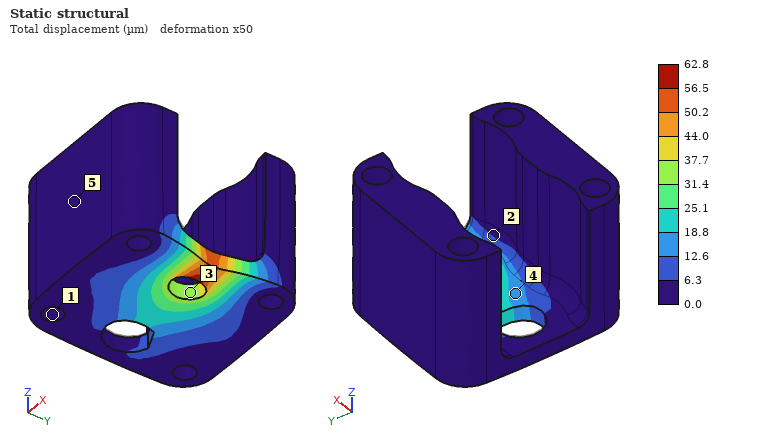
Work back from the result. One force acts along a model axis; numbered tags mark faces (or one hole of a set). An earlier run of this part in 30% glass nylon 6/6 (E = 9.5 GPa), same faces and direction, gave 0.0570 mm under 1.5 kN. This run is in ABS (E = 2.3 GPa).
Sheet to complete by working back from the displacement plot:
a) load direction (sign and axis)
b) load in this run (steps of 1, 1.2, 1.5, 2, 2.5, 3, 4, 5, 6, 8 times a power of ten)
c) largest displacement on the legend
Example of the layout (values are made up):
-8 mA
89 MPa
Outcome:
-X
400 N
62.8 µm
